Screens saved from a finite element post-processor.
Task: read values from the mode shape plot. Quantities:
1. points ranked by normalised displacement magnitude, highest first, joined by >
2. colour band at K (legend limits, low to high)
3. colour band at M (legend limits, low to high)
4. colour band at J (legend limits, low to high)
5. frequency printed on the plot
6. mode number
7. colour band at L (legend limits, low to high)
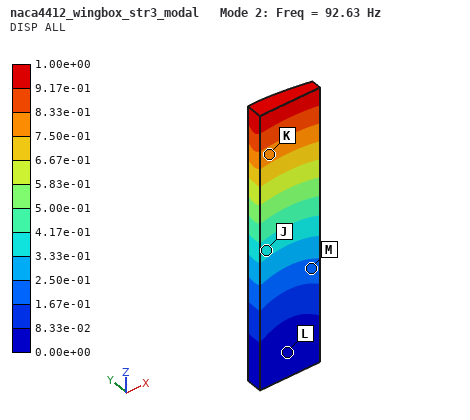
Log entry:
K > J > M > L
7.50e-01 to 8.33e-01
1.67e-01 to 2.50e-01
3.33e-01 to 4.17e-01
92.63 Hz
2
0.00e+00 to 8.33e-02
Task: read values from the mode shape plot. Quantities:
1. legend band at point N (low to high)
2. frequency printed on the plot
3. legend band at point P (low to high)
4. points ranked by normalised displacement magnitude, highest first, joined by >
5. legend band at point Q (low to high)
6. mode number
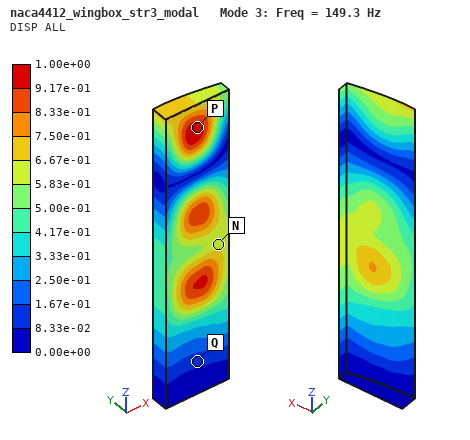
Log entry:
5.83e-01 to 6.67e-01
149.3 Hz
9.17e-01 to 1.00e+00
P > N > Q
8.33e-02 to 1.67e-01
3
